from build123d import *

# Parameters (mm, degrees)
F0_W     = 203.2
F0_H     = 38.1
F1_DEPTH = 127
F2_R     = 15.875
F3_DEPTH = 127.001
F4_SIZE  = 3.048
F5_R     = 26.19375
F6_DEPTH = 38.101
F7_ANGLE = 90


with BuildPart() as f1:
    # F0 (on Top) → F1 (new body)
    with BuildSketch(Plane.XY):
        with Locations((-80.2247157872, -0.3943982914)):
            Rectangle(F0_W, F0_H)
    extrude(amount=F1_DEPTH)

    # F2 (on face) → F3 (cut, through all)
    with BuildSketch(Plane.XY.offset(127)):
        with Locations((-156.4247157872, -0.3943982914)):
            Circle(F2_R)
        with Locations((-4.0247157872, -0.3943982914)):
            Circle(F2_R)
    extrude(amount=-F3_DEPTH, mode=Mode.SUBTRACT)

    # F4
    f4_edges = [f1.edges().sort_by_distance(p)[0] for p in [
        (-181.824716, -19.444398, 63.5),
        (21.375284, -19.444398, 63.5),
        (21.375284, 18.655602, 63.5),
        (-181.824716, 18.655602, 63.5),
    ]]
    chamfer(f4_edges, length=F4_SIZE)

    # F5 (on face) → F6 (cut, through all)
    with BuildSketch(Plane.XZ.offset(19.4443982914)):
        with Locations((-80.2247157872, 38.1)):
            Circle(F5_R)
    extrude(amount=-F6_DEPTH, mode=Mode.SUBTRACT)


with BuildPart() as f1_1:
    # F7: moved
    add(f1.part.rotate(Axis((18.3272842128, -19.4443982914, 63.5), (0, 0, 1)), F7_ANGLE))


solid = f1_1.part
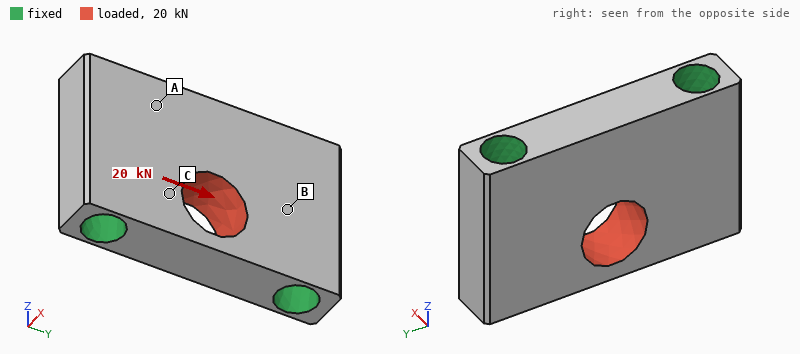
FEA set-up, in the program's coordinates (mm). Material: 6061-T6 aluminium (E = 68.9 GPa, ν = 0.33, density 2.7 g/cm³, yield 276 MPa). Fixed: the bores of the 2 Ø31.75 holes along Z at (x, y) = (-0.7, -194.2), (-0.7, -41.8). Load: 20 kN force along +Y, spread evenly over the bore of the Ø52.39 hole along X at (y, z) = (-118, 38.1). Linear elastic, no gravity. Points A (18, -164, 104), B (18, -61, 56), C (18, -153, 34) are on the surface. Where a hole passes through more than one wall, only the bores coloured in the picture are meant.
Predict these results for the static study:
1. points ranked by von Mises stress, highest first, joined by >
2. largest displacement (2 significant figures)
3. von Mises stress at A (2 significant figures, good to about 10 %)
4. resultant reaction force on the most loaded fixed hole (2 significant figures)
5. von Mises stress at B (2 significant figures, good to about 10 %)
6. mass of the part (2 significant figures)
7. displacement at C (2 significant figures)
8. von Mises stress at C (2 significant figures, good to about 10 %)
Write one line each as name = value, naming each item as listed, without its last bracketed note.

points ranked by von Mises stress, highest first, joined by > = C > B > A
largest displacement = 3.4 µm
von Mises stress at A = 0.76 MPa
resultant reaction force on the most loaded fixed hole = 10 kN
von Mises stress at B = 1.7 MPa
mass of the part = 1.9 kg
displacement at C = 1.3 µm
von Mises stress at C = 3.2 MPa
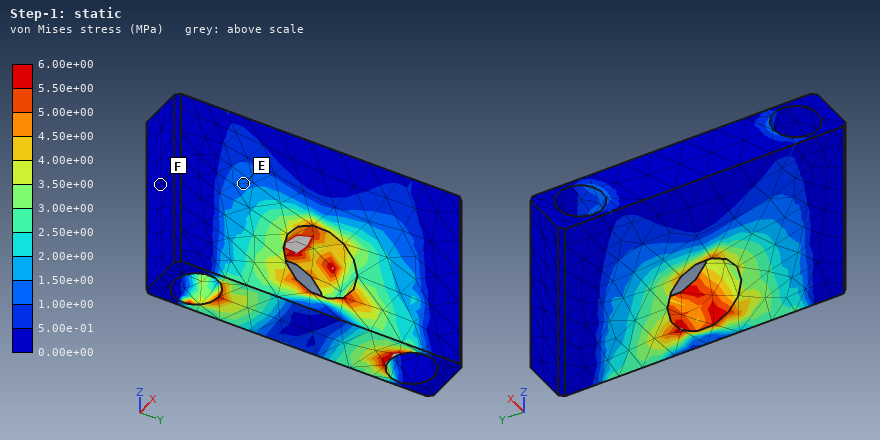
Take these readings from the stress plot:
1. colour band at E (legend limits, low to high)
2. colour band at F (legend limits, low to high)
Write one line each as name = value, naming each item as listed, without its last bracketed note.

colour band at E = 1.00e+00 to 1.50e+00 MPa
colour band at F = 0.00e+00 to 5.00e-01 MPa
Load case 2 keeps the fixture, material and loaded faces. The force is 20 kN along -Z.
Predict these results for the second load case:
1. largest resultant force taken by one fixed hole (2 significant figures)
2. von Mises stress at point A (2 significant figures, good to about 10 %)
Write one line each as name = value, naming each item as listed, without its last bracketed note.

largest resultant force taken by one fixed hole = 10 kN
von Mises stress at point A = 3.0 MPa
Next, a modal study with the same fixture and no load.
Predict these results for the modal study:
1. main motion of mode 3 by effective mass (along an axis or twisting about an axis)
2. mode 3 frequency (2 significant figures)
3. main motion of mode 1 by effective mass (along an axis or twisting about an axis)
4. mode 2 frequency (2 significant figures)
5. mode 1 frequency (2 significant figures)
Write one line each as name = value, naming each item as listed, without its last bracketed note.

main motion of mode 3 by effective mass = along Z
mode 3 frequency = 12 kHz
main motion of mode 1 by effective mass = along X
mode 2 frequency = 9700 Hz
mode 1 frequency = 8300 Hz
